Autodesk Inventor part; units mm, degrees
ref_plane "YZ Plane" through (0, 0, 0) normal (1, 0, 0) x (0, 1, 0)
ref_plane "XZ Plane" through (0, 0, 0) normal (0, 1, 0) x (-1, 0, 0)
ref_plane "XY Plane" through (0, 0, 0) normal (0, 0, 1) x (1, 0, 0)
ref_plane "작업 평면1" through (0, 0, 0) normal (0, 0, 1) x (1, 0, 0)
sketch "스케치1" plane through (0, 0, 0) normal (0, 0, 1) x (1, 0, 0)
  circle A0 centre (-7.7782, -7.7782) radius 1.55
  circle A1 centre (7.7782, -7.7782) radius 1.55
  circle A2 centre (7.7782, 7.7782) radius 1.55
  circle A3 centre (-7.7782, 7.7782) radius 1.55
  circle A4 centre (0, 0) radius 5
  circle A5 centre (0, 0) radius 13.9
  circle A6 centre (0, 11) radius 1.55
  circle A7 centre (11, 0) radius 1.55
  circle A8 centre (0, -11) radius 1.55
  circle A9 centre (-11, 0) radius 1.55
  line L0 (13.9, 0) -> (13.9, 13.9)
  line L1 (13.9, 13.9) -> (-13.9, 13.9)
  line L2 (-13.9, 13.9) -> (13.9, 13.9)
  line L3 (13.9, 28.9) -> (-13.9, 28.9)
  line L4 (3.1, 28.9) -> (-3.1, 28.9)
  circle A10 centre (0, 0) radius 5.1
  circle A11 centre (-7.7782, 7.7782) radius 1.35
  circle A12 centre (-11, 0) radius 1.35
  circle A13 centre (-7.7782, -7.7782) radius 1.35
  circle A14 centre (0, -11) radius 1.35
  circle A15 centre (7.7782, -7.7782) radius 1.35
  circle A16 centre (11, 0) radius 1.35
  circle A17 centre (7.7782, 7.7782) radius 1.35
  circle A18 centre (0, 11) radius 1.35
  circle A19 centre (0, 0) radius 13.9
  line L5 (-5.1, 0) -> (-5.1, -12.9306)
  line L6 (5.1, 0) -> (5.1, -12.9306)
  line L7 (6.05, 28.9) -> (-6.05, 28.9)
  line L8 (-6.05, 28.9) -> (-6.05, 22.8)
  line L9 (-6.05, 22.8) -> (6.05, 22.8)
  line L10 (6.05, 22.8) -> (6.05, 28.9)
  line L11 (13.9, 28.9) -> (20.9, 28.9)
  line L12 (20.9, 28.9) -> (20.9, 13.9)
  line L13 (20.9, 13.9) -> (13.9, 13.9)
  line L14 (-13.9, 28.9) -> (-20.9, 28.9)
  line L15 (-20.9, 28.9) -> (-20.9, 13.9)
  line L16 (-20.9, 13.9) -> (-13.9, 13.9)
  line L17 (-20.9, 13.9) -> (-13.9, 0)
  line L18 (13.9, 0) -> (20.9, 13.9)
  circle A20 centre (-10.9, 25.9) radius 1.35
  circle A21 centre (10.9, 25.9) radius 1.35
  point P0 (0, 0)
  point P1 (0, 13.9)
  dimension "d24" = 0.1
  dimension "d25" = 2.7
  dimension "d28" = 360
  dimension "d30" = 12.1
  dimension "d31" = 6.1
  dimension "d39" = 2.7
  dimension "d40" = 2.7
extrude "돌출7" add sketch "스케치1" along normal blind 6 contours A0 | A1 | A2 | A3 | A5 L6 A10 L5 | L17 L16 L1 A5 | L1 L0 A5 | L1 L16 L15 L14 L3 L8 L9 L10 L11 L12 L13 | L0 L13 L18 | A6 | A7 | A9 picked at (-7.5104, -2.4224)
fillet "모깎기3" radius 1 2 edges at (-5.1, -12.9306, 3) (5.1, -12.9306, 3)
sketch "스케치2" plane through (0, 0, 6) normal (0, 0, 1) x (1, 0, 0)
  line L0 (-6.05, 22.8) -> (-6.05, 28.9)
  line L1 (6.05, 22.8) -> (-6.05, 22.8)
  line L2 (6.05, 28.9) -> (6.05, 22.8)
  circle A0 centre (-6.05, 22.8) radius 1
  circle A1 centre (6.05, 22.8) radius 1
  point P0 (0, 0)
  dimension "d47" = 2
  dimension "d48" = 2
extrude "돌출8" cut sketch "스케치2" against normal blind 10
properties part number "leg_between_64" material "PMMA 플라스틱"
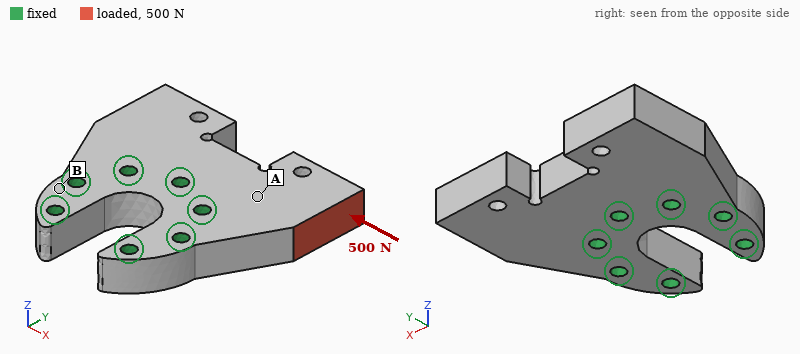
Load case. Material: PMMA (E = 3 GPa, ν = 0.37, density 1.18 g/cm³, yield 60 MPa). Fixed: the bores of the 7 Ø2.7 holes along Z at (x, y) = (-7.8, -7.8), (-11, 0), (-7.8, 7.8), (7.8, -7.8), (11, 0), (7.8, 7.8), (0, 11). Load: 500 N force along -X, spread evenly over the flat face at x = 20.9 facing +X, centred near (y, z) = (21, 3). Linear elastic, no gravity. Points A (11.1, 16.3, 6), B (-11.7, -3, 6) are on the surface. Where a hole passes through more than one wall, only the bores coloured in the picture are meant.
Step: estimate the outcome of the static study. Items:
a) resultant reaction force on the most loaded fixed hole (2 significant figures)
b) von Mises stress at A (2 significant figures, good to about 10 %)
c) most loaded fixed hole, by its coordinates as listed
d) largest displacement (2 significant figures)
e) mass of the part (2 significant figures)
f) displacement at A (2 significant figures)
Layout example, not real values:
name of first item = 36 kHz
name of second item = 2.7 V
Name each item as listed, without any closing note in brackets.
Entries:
resultant reaction force on the most loaded fixed hole = 370 N
von Mises stress at A = 6.5 MPa
most loaded fixed hole, by its coordinates as listed = (0, 11)
largest displacement = 0.17 mm
mass of the part = 7.8 g
displacement at A = 0.041 mm
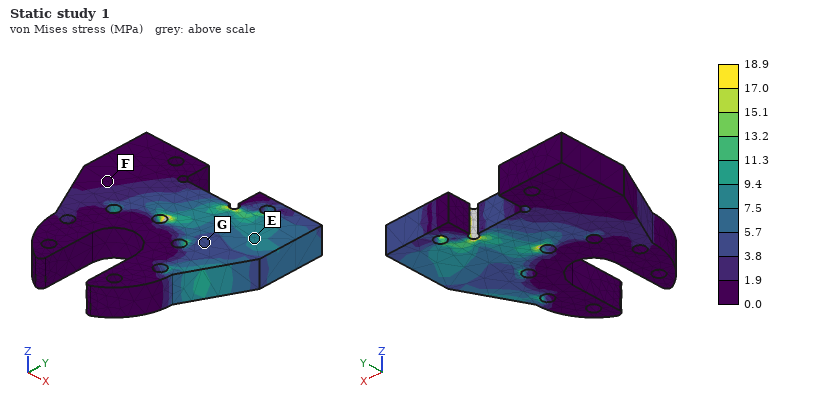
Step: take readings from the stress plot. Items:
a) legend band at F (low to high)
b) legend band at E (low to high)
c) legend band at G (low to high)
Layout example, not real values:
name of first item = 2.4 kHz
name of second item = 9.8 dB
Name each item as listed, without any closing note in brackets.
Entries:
legend band at F = 0.0 to 1.9 MPa
legend band at E = 7.5 to 9.4 MPa
legend band at G = 3.8 to 5.7 MPa
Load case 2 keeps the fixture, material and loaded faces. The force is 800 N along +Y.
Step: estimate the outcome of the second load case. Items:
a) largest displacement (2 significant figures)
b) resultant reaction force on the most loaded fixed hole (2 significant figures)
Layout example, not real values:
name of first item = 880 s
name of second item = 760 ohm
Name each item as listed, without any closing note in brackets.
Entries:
largest displacement = 0.37 mm
resultant reaction force on the most loaded fixed hole = 590 N
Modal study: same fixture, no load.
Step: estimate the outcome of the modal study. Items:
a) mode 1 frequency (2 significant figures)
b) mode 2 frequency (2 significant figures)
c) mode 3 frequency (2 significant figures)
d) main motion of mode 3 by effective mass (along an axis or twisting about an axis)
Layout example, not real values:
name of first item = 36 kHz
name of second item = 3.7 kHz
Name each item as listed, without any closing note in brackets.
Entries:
mode 1 frequency = 3500 Hz
mode 2 frequency = 3500 Hz
mode 3 frequency = 7300 Hz
main motion of mode 3 by effective mass = along X
